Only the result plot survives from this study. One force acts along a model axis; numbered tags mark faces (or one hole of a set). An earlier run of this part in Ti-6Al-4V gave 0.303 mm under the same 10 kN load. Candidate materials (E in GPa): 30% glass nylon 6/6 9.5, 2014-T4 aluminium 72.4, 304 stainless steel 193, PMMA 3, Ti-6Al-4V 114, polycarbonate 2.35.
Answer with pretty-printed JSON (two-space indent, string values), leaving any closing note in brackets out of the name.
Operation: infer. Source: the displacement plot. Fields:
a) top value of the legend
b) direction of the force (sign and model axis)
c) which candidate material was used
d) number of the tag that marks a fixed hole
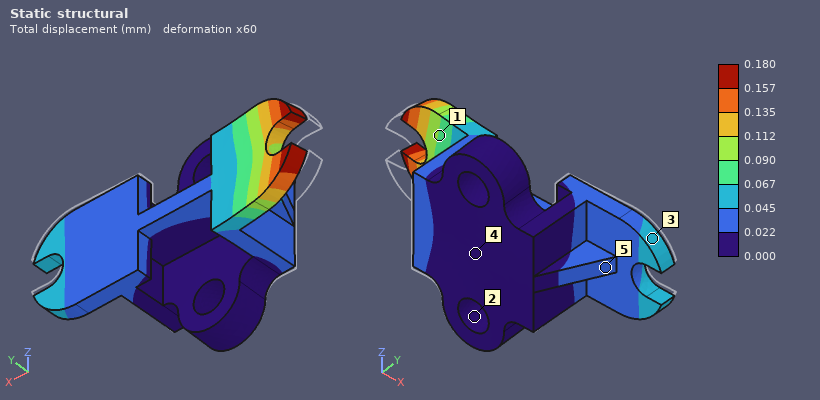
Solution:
{
  "top value of the legend": "0.180 mm",
  "direction of the force": "+Y",
  "which candidate material was used": "304 stainless steel",
  "number of the tag that marks a fixed hole": "2"
}
